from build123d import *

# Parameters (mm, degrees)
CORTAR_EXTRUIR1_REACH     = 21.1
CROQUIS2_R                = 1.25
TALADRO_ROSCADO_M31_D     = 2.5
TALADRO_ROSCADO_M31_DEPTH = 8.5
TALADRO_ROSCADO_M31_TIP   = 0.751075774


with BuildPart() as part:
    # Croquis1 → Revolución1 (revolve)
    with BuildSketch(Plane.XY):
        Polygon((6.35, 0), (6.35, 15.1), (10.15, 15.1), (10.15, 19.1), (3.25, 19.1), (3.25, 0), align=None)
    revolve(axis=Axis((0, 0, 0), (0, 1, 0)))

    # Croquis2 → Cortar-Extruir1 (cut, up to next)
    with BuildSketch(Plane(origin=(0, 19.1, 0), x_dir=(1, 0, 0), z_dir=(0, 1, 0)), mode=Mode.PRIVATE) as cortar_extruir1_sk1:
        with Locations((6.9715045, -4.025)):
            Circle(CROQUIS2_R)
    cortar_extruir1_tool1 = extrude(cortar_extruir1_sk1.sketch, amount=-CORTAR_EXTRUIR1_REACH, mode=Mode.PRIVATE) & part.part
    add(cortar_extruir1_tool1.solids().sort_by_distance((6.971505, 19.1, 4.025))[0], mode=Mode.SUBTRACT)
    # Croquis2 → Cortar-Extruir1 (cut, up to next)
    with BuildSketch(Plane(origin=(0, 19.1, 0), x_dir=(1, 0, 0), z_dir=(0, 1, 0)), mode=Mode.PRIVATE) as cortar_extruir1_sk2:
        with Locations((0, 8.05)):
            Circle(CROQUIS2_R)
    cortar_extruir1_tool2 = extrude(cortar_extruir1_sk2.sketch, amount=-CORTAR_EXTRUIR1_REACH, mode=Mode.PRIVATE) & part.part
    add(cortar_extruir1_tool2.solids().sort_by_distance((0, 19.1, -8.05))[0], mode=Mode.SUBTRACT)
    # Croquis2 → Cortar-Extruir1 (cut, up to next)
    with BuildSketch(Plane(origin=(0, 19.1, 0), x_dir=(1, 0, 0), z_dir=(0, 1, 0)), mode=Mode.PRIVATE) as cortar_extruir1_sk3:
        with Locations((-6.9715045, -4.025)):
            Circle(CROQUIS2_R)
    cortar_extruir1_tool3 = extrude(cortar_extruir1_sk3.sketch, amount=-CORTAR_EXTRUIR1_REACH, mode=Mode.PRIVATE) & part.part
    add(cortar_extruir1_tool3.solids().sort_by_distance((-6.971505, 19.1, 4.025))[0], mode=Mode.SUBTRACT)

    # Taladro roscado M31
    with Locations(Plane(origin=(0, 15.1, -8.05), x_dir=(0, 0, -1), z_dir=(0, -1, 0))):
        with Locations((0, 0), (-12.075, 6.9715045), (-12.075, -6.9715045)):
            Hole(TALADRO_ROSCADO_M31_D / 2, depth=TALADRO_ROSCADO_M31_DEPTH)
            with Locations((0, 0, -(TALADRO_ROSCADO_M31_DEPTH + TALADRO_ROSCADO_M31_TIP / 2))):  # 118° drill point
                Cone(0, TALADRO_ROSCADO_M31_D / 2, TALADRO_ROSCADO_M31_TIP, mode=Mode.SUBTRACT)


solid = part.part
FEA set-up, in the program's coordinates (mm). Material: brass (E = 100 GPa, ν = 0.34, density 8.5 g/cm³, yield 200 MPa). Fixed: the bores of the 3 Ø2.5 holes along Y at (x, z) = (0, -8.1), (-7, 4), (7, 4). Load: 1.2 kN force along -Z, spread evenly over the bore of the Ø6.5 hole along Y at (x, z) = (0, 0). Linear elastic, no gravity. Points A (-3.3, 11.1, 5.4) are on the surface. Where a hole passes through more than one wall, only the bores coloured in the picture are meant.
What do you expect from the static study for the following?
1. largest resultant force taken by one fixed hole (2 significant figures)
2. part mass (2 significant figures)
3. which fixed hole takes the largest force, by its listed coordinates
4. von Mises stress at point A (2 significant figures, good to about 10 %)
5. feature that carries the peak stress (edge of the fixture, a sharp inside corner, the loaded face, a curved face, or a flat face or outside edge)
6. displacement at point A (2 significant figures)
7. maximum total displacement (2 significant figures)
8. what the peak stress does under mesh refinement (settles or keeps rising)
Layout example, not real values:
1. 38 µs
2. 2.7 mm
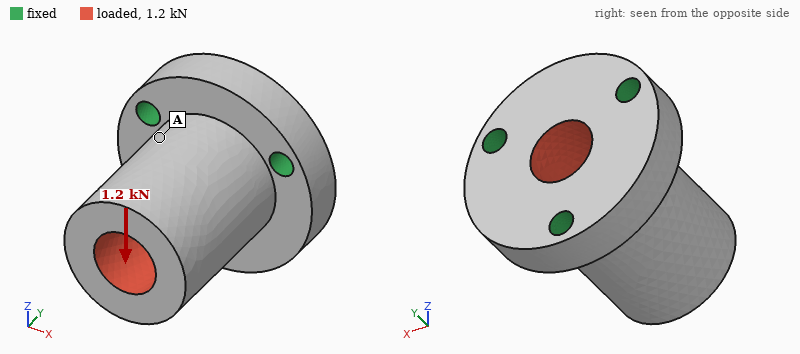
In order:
1. 840 N
2. 21 g
3. (0, -8.1)
4. 16 MPa
5. a sharp inside corner
6. 5.6 µm
7. 14 µm
8. keeps rising
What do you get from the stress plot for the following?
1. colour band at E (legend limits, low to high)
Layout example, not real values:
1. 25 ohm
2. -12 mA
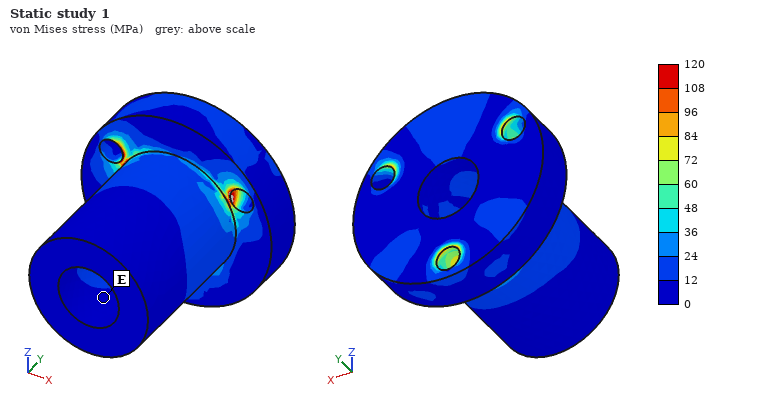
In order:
1. 0 to 12 MPa
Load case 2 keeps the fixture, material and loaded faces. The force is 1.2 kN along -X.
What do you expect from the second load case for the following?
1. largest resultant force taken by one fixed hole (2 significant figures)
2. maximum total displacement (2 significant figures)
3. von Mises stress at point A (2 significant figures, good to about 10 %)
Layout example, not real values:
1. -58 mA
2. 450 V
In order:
1. 750 N
2. 14 µm
3. 20 MPa
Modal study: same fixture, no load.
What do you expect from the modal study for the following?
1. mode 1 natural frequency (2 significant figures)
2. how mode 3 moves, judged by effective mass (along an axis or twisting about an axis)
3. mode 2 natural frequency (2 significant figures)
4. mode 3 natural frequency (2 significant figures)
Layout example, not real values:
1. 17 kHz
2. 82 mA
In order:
1. 14 kHz
2. twisting about Y
3. 14 kHz
4. 31 kHz
